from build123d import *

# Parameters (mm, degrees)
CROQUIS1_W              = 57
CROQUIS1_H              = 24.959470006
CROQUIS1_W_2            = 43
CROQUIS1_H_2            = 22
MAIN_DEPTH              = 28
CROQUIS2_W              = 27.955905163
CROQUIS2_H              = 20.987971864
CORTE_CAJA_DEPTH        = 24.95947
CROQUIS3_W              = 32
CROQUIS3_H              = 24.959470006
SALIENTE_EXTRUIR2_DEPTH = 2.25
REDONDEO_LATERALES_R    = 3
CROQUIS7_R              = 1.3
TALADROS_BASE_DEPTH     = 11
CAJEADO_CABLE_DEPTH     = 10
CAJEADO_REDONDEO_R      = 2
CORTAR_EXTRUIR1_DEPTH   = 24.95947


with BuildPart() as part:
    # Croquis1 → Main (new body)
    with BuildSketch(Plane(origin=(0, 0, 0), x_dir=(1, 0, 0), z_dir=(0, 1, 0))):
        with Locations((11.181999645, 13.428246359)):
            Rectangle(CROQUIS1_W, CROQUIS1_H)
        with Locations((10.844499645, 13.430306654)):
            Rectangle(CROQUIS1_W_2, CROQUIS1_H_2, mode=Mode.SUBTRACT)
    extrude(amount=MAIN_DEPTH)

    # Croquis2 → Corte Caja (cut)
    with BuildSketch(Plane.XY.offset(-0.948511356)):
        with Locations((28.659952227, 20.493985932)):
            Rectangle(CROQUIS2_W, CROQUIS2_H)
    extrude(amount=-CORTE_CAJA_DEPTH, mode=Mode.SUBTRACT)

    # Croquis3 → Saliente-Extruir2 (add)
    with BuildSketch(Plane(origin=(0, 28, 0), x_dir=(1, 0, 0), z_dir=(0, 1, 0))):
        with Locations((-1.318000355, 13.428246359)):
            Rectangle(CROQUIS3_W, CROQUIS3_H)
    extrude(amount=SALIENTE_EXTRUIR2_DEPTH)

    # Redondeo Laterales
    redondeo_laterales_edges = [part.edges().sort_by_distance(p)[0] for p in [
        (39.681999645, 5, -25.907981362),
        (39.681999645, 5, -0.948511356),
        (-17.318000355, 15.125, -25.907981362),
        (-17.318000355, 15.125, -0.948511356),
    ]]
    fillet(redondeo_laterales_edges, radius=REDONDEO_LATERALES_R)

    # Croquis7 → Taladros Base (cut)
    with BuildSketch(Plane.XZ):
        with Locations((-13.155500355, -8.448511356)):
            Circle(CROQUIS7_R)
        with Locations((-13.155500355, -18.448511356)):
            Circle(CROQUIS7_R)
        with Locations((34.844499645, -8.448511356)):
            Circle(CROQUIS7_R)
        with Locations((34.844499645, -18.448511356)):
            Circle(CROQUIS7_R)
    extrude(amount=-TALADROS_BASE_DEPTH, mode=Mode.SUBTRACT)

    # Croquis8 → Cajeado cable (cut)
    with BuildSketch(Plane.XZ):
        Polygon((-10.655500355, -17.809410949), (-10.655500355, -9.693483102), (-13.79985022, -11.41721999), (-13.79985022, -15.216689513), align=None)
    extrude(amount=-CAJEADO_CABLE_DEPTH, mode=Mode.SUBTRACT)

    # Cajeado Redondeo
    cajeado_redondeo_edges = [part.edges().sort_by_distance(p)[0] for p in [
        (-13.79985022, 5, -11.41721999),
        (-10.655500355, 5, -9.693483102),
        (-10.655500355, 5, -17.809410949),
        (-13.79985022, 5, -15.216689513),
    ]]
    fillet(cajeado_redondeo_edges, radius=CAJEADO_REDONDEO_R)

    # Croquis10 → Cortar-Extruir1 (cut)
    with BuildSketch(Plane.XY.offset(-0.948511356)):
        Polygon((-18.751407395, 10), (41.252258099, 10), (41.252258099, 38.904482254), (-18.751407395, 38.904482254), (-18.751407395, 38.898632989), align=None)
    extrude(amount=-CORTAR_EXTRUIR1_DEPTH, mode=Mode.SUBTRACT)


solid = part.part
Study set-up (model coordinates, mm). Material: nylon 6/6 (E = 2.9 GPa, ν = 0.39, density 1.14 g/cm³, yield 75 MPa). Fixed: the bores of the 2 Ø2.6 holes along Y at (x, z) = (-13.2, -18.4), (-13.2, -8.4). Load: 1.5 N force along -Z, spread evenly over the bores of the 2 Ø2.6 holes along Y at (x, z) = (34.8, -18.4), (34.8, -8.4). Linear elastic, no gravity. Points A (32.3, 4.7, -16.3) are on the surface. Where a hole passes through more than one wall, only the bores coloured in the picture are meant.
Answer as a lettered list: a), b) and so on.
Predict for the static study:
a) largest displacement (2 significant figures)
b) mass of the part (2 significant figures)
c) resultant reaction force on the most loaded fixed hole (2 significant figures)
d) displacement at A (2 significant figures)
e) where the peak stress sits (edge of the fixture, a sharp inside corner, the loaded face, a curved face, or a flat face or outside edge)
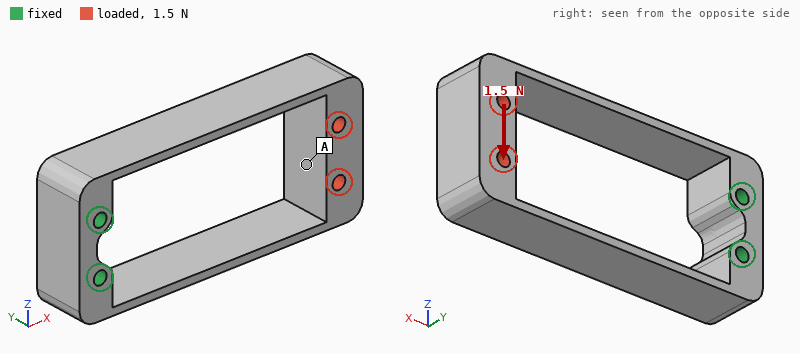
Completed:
a) 0.68 mm
b) 4.9 g
c) 3.2 N
d) 0.68 mm
e) a flat face or outside edge
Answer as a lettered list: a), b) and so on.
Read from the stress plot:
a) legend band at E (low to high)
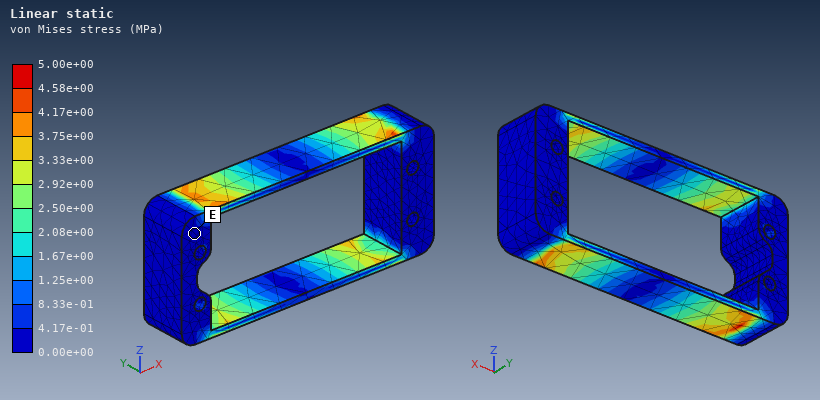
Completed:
a) 0.00e+00 to 4.17e-01 MPa
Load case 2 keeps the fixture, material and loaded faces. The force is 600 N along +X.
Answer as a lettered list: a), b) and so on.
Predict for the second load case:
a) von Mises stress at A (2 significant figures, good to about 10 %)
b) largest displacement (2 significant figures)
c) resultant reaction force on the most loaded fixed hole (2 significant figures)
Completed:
a) 29 MPa
b) 0.60 mm
c) 370 N
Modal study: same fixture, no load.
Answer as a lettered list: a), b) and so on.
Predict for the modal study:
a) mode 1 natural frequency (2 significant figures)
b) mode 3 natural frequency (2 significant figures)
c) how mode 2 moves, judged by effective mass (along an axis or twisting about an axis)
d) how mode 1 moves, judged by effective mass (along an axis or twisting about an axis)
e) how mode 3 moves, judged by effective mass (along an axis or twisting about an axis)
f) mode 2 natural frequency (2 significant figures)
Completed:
a) 150 Hz
b) 960 Hz
c) along Y
d) along Z
e) twisting about X
f) 400 Hz
